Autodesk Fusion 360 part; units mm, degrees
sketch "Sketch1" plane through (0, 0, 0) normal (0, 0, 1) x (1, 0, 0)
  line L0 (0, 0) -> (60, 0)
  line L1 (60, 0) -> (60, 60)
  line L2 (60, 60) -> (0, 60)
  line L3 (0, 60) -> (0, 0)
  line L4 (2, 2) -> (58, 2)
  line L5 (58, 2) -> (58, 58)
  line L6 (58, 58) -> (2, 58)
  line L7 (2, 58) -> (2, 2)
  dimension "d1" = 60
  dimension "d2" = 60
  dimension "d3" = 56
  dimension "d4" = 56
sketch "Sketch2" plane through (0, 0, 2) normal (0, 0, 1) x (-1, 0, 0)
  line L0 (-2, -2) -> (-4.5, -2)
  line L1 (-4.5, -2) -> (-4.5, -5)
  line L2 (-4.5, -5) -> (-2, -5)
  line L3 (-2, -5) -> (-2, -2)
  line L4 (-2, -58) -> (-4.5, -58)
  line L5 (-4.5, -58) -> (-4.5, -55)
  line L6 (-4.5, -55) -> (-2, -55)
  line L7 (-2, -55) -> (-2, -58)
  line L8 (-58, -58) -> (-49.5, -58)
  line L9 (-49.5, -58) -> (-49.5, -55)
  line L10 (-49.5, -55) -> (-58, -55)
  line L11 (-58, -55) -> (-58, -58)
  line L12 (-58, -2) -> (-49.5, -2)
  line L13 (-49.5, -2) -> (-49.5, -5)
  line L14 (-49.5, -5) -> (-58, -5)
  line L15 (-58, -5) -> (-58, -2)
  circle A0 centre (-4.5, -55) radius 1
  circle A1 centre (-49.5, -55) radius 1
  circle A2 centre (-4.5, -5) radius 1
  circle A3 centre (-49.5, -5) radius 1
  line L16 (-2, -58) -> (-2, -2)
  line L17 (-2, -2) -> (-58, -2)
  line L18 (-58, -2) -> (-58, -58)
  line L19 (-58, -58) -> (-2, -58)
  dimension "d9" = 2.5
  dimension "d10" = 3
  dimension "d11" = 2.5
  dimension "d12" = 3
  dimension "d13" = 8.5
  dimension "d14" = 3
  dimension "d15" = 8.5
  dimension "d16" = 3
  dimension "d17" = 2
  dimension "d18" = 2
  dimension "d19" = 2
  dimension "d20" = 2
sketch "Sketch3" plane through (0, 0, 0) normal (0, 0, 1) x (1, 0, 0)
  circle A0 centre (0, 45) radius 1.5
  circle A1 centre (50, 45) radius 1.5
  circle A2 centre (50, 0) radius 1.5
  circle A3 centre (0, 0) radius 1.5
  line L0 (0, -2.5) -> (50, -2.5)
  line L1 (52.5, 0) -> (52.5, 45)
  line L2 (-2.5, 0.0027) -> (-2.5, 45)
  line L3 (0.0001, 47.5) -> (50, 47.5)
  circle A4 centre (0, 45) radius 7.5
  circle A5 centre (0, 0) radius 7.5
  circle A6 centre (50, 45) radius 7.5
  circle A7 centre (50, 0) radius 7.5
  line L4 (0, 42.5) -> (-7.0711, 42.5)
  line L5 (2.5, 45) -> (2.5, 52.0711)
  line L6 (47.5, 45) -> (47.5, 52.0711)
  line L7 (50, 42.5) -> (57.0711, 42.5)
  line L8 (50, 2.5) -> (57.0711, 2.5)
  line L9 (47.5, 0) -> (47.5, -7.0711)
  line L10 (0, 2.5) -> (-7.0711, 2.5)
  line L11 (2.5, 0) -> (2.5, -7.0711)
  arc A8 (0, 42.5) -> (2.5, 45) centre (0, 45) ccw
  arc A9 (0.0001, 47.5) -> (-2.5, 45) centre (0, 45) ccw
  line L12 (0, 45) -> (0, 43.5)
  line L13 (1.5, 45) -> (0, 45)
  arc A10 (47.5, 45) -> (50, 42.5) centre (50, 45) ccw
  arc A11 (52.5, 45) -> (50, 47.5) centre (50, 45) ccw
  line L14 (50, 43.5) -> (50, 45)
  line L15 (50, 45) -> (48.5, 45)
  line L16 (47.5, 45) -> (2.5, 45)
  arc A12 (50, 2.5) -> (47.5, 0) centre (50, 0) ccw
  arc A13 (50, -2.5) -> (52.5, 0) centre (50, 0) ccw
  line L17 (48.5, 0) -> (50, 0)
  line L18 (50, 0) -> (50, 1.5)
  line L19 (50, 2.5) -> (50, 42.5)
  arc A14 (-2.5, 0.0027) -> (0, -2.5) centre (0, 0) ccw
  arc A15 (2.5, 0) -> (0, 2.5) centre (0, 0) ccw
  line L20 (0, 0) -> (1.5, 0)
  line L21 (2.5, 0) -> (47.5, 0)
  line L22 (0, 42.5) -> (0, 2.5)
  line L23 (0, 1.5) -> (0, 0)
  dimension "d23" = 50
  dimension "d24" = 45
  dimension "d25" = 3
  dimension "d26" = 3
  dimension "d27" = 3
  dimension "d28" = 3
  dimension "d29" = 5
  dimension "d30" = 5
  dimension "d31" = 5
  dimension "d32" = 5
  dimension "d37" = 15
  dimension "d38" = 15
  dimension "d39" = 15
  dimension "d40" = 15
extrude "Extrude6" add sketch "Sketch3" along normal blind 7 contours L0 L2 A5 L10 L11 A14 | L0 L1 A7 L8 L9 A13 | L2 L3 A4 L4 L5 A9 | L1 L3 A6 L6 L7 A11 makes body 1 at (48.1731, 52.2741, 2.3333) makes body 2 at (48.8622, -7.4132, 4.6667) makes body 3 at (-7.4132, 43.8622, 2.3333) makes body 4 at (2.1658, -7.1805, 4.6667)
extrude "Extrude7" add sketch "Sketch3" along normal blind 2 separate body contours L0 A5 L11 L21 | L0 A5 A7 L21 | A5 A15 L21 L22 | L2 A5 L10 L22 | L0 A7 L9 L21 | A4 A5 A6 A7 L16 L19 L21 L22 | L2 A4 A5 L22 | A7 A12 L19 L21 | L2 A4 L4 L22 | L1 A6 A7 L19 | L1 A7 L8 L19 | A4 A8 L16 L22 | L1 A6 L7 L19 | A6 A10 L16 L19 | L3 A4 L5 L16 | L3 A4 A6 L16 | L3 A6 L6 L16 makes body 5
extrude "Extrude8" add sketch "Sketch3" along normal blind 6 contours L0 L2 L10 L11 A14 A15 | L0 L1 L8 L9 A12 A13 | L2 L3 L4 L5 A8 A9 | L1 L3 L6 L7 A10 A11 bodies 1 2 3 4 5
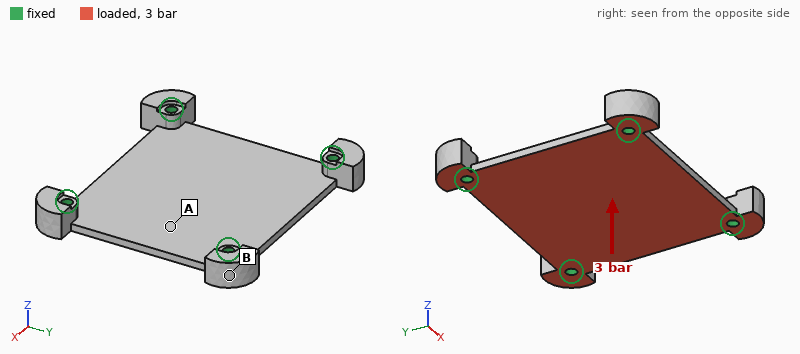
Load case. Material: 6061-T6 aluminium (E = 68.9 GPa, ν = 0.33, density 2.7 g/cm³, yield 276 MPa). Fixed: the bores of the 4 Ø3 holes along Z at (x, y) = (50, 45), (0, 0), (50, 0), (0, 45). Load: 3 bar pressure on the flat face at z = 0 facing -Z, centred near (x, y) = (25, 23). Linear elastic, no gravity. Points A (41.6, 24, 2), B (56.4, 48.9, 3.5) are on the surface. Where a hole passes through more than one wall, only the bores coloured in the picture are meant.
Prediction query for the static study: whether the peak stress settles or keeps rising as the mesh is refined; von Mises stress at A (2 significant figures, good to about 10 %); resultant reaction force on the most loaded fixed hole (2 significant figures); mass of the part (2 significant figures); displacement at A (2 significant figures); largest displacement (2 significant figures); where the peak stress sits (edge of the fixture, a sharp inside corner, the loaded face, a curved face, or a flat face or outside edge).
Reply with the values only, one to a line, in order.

keeps rising
45 MPa
230 N
20 g
0.15 mm
0.22 mm
edge of the fixture
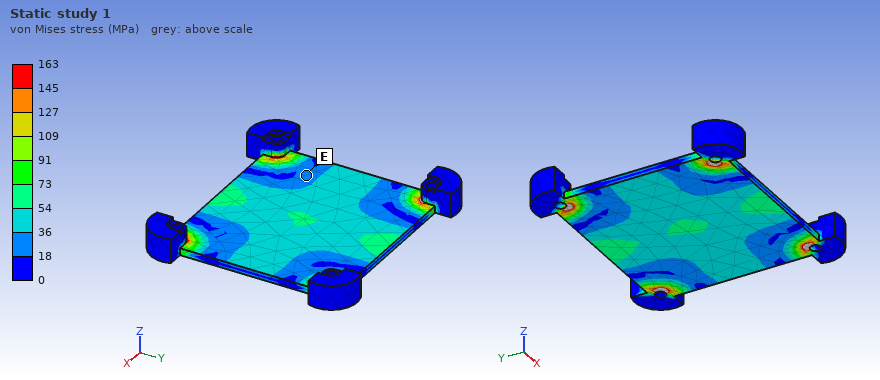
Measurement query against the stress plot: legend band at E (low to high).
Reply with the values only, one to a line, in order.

18 to 36 MPa
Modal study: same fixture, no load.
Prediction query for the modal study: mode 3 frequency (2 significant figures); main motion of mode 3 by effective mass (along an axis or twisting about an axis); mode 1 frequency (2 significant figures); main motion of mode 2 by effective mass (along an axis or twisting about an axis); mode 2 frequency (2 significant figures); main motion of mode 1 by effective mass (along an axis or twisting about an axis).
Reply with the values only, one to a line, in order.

5800 Hz
twisting about Y
3100 Hz
twisting about X
5100 Hz
along Z
